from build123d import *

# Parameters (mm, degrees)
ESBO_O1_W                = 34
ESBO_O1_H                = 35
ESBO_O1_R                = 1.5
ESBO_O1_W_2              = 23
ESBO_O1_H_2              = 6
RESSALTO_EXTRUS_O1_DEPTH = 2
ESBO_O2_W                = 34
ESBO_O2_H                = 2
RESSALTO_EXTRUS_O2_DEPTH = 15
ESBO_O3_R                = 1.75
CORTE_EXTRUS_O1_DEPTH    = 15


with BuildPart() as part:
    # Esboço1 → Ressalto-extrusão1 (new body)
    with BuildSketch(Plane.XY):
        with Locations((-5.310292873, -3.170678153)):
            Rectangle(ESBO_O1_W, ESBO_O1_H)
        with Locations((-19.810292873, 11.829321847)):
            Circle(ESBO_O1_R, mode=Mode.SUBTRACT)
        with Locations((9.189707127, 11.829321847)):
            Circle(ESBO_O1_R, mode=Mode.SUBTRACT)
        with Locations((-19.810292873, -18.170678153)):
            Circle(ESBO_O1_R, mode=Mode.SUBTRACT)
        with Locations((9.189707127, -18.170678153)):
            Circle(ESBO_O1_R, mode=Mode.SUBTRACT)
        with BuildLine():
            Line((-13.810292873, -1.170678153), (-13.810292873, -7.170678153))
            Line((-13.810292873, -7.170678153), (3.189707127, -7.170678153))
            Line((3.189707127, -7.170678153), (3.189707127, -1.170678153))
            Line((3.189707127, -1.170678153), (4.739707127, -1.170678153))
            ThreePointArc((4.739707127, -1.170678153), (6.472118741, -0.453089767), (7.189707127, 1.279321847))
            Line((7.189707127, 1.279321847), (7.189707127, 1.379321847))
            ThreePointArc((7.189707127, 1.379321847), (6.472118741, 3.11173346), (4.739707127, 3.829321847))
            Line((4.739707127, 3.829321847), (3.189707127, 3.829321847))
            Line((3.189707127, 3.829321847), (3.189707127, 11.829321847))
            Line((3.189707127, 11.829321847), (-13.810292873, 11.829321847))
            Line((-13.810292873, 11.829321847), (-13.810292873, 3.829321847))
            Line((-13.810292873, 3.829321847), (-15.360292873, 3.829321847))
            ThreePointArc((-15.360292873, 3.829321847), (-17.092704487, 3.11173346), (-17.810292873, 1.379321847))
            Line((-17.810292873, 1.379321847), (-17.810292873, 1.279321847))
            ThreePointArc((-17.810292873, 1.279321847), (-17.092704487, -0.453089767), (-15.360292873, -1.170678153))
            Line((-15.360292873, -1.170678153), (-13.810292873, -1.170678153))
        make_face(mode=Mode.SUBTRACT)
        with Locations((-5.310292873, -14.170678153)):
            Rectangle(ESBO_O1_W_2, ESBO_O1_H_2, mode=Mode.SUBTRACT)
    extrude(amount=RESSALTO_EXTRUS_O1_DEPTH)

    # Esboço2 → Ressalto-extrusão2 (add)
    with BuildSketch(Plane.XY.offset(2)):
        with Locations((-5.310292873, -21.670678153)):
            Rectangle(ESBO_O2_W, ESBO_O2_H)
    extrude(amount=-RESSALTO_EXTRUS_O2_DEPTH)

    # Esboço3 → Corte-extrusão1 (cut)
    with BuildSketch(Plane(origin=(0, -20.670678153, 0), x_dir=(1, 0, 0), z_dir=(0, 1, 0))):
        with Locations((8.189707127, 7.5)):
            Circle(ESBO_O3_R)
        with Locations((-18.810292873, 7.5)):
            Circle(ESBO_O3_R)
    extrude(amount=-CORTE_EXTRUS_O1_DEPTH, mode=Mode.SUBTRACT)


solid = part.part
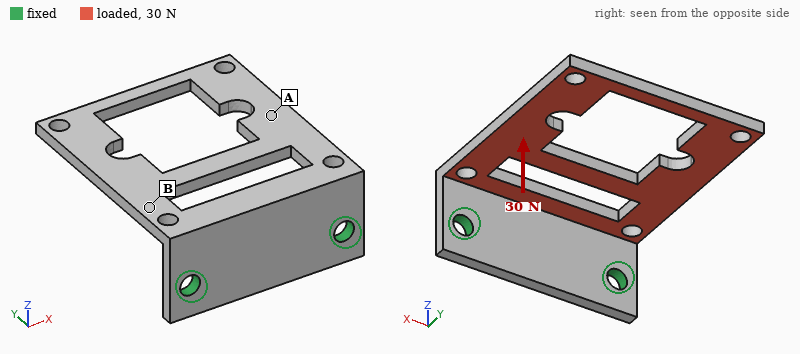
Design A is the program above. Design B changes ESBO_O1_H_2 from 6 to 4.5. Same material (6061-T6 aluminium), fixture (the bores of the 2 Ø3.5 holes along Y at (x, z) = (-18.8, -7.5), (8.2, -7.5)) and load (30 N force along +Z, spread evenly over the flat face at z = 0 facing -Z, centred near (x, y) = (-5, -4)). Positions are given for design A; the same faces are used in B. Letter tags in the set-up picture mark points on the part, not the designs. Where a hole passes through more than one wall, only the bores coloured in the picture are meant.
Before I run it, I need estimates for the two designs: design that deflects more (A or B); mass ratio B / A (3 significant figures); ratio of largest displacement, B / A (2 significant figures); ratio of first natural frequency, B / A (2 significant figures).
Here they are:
A
1.03
0.89
1.0
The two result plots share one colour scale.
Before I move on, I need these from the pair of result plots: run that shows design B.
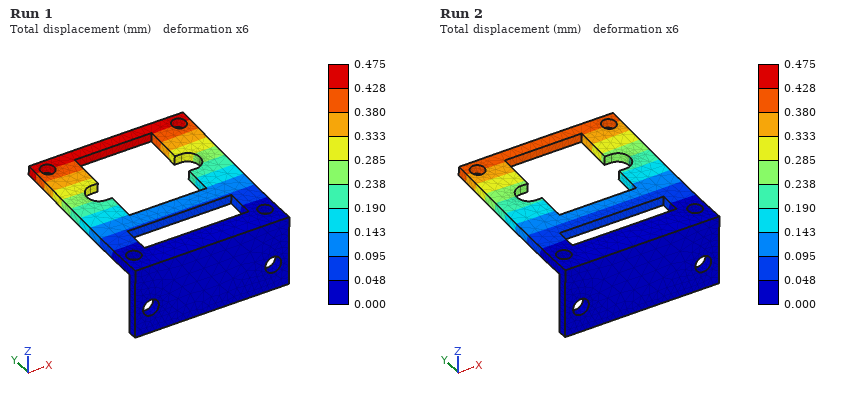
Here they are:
Run 2
